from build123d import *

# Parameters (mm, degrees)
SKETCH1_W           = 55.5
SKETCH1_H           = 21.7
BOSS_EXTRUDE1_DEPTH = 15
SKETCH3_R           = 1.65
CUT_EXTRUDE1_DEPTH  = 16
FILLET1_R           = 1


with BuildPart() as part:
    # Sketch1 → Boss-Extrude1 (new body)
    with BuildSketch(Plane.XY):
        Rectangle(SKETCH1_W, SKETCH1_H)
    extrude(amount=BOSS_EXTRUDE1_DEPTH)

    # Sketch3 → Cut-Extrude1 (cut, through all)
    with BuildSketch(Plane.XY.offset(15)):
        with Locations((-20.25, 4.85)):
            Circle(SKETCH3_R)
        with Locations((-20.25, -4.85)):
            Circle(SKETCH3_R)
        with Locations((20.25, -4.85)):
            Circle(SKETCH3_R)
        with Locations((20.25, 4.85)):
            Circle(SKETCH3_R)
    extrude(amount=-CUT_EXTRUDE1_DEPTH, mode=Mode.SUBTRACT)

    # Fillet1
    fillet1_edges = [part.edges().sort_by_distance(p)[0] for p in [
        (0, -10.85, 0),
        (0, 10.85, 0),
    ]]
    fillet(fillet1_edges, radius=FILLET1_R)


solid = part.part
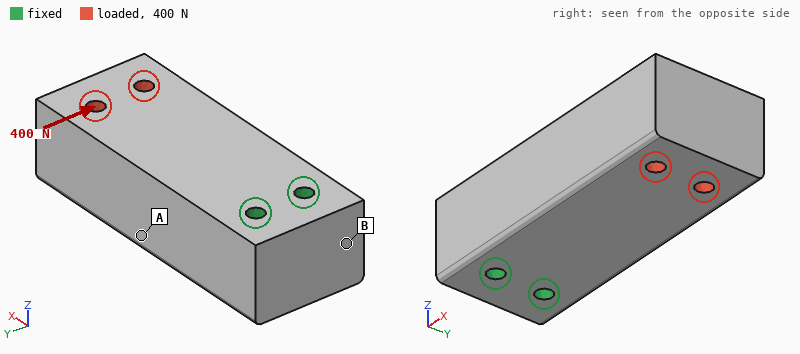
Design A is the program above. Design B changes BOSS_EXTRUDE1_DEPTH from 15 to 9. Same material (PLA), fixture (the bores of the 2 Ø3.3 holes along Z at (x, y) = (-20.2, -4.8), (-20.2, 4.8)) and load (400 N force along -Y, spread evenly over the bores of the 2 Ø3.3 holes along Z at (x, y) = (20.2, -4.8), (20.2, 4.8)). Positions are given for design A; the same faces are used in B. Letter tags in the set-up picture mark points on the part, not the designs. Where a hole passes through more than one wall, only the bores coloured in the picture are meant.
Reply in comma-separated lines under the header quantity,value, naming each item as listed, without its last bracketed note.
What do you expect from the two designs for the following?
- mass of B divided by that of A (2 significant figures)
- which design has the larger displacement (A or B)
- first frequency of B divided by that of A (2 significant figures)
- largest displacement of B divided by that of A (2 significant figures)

quantity,value
mass of B divided by that of A,0.60
which design has the larger displacement,B
first frequency of B divided by that of A,0.64
largest displacement of B divided by that of A,1.7
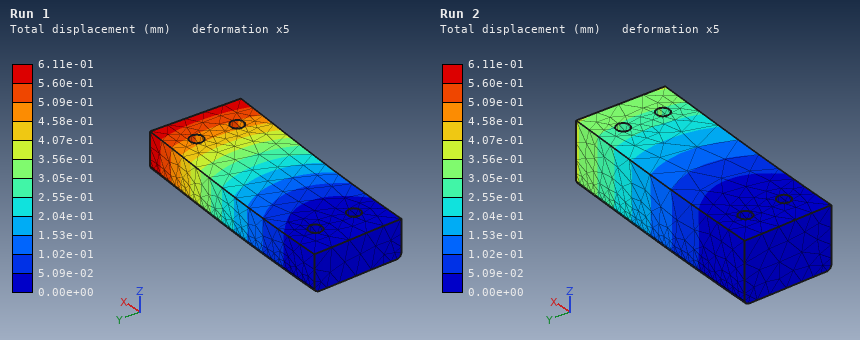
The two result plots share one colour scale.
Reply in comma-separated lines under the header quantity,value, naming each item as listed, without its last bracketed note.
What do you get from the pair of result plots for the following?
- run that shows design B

quantity,value
run that shows design B,Run 1
